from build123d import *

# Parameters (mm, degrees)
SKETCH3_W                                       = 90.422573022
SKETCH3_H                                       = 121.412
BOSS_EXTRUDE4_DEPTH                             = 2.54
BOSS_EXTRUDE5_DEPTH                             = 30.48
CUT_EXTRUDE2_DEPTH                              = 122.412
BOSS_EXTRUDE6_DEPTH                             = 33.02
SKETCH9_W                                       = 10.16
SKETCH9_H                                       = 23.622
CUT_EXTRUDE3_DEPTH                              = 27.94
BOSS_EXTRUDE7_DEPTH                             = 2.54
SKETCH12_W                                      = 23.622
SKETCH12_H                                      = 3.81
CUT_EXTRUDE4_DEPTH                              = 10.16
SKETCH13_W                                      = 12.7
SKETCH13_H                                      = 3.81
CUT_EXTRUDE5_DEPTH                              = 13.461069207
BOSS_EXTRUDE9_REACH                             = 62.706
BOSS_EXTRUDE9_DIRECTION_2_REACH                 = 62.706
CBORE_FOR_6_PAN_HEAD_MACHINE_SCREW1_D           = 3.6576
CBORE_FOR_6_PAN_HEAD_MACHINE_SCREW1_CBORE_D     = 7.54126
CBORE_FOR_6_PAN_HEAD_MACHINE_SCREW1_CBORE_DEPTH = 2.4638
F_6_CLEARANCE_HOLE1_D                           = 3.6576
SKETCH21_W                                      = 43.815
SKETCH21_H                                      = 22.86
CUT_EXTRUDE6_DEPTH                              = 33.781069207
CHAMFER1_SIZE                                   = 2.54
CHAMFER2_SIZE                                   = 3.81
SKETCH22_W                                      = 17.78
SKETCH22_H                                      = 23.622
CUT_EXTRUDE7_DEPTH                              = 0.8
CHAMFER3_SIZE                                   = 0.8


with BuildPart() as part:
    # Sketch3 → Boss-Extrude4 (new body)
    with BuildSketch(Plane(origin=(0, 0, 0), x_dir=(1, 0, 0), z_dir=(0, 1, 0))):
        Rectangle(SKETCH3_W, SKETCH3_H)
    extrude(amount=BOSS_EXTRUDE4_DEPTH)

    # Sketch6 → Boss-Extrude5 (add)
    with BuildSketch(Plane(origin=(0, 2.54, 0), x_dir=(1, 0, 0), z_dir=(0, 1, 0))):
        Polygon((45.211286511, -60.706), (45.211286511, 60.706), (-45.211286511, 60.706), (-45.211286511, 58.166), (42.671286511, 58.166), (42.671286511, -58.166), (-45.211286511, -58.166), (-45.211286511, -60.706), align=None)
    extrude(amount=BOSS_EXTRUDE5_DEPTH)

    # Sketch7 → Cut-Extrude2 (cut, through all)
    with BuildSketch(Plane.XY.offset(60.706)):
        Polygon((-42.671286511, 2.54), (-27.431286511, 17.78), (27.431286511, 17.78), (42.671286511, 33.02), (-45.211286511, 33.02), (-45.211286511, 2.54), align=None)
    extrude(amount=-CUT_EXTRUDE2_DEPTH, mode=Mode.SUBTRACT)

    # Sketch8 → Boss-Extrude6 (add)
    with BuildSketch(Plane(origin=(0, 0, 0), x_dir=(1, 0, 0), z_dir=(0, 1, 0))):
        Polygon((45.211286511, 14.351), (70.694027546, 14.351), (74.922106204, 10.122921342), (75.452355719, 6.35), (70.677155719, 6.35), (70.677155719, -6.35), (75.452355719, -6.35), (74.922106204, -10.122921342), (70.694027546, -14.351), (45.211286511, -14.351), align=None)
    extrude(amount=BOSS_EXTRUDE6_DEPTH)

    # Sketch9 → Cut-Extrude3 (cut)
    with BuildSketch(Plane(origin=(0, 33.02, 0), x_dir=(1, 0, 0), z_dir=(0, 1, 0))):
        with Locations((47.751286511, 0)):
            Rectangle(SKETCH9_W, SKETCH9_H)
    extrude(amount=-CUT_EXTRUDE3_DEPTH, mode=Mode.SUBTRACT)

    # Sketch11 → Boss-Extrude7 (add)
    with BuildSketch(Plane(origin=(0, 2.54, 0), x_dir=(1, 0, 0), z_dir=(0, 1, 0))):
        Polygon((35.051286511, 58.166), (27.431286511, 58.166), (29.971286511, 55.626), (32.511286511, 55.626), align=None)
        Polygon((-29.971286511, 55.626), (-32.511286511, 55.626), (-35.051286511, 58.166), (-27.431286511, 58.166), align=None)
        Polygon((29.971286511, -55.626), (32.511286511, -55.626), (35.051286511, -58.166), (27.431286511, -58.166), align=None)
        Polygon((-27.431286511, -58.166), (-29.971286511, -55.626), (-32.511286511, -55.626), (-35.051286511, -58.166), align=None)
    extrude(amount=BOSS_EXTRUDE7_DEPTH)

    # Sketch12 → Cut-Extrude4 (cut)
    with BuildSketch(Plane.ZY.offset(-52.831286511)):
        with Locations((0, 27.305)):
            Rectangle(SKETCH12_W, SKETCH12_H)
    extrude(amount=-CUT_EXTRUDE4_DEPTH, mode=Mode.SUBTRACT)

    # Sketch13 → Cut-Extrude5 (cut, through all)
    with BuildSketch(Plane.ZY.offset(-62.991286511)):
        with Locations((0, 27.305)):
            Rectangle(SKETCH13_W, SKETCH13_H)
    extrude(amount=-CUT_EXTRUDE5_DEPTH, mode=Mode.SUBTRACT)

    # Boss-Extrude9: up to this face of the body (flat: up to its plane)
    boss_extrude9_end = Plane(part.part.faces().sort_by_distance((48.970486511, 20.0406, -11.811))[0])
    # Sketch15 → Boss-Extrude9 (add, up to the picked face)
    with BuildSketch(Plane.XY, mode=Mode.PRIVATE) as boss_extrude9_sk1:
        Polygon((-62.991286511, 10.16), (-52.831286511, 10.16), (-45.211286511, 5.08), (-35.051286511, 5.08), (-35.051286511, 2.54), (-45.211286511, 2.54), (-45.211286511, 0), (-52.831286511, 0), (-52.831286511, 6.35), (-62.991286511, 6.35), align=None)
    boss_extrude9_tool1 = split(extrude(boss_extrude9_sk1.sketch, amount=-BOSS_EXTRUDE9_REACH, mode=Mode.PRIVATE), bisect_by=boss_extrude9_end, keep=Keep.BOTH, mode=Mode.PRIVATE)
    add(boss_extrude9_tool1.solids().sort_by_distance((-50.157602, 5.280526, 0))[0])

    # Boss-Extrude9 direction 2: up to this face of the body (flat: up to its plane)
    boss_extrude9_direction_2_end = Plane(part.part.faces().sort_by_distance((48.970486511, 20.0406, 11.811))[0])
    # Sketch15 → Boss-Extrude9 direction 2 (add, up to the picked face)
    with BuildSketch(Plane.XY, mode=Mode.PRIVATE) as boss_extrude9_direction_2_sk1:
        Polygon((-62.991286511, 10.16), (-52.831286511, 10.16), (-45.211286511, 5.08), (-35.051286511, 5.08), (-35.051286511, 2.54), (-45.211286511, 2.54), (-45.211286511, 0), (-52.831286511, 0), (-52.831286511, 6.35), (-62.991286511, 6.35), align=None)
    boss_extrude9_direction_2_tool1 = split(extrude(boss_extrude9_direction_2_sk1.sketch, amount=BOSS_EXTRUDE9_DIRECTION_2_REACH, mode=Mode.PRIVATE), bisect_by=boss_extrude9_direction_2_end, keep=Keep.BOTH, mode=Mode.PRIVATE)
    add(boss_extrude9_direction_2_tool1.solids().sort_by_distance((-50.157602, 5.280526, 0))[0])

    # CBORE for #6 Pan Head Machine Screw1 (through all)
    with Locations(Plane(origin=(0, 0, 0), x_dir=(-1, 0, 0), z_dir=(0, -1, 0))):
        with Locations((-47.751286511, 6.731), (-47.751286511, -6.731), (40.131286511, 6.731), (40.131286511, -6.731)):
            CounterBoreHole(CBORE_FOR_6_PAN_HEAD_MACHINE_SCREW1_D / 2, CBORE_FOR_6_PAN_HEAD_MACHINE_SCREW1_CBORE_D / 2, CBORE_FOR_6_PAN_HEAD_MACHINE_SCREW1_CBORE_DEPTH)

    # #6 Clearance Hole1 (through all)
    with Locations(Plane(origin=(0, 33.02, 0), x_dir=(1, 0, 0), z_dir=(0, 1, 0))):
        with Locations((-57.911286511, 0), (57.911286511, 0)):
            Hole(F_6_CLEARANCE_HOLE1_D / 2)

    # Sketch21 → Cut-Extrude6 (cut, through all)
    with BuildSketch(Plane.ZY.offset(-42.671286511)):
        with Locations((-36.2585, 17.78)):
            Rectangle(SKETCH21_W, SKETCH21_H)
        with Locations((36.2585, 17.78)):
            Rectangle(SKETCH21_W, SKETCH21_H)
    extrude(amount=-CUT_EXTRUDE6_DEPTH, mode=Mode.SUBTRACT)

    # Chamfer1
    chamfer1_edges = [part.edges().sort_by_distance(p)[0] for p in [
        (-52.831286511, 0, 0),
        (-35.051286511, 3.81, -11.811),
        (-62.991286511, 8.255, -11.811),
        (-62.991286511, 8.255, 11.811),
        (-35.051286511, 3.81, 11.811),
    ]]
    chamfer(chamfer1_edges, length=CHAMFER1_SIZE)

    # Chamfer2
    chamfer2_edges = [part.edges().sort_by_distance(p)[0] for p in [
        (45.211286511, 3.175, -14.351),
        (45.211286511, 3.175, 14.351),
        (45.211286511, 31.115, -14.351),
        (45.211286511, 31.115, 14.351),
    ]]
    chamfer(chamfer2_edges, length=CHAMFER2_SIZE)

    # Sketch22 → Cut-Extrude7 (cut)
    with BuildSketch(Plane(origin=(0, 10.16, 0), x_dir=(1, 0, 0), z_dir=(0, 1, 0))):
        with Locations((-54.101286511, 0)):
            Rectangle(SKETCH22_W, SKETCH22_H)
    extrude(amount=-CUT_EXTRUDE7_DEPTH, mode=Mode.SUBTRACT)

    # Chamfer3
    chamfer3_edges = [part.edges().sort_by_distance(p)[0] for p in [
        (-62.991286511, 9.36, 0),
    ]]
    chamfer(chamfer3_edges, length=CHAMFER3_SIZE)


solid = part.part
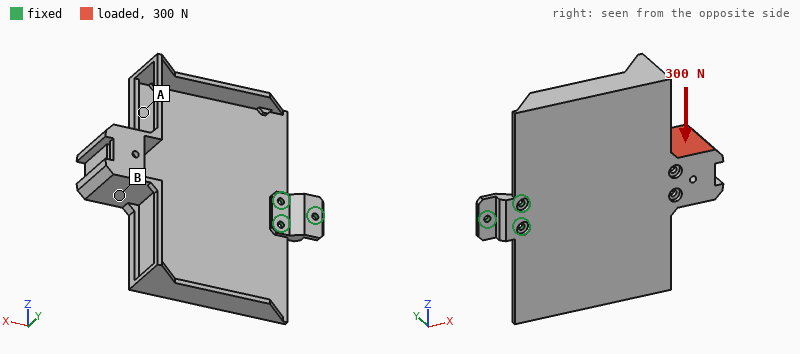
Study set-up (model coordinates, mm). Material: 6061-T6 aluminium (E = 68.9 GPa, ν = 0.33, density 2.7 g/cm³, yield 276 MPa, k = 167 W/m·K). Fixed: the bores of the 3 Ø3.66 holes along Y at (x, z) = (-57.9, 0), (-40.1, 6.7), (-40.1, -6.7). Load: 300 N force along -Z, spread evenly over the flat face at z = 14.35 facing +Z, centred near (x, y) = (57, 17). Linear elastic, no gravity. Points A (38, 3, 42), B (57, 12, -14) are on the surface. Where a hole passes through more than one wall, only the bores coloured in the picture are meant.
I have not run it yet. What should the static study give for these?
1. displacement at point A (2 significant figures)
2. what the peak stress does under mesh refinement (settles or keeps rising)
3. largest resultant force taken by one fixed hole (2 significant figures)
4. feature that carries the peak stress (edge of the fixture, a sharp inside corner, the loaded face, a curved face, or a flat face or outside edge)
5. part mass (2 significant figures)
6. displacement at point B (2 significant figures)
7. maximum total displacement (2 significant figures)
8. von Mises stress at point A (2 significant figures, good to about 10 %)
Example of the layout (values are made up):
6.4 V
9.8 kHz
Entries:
0.89 mm
keeps rising
1.2 kN
edge of the fixture
160 g
0.51 mm
1.6 mm
17 MPa
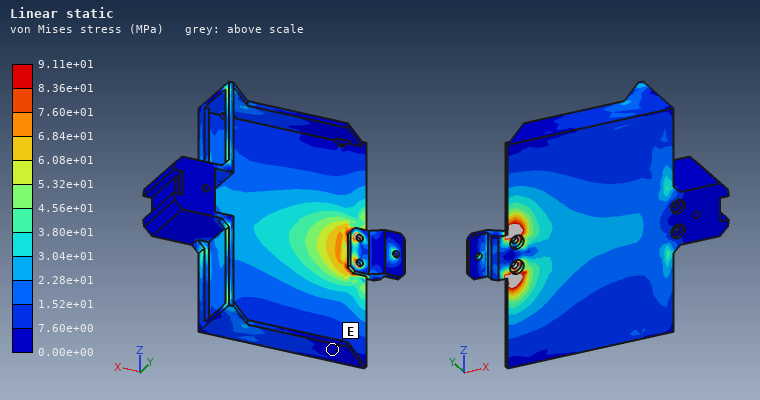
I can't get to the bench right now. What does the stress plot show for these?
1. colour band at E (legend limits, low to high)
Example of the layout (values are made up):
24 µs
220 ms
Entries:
0.00e+00 to 7.60e+00 MPa
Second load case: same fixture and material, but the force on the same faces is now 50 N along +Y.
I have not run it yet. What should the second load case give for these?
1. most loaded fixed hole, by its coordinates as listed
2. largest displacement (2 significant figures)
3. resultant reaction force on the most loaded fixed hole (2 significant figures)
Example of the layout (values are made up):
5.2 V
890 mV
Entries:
(-57.9, 0)
2.0 mm
250 N
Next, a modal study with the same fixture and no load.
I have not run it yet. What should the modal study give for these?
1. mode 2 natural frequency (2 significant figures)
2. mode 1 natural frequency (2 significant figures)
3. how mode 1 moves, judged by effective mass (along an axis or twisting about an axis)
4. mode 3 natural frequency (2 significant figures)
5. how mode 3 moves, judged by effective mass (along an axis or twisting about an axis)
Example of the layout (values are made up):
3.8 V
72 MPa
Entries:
210 Hz
100 Hz
along Y
550 Hz
along Y
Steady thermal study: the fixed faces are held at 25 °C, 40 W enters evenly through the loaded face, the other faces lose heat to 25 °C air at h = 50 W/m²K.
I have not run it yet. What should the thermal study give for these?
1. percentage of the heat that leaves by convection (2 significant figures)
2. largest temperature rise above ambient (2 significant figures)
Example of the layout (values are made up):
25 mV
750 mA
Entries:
84 %
53 K
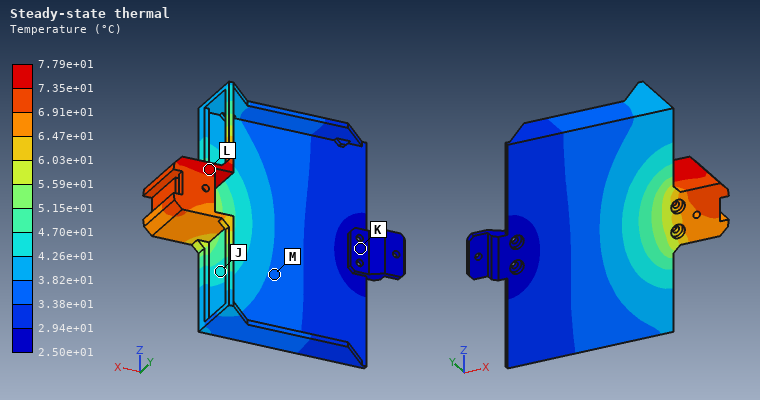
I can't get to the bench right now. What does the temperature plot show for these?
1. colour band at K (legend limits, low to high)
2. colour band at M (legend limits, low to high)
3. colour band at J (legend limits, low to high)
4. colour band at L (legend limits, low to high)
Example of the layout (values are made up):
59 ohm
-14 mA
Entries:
2.50e+01 to 2.94e+01 °C
3.38e+01 to 3.82e+01 °C
4.26e+01 to 4.70e+01 °C
7.35e+01 to 7.79e+01 °C
